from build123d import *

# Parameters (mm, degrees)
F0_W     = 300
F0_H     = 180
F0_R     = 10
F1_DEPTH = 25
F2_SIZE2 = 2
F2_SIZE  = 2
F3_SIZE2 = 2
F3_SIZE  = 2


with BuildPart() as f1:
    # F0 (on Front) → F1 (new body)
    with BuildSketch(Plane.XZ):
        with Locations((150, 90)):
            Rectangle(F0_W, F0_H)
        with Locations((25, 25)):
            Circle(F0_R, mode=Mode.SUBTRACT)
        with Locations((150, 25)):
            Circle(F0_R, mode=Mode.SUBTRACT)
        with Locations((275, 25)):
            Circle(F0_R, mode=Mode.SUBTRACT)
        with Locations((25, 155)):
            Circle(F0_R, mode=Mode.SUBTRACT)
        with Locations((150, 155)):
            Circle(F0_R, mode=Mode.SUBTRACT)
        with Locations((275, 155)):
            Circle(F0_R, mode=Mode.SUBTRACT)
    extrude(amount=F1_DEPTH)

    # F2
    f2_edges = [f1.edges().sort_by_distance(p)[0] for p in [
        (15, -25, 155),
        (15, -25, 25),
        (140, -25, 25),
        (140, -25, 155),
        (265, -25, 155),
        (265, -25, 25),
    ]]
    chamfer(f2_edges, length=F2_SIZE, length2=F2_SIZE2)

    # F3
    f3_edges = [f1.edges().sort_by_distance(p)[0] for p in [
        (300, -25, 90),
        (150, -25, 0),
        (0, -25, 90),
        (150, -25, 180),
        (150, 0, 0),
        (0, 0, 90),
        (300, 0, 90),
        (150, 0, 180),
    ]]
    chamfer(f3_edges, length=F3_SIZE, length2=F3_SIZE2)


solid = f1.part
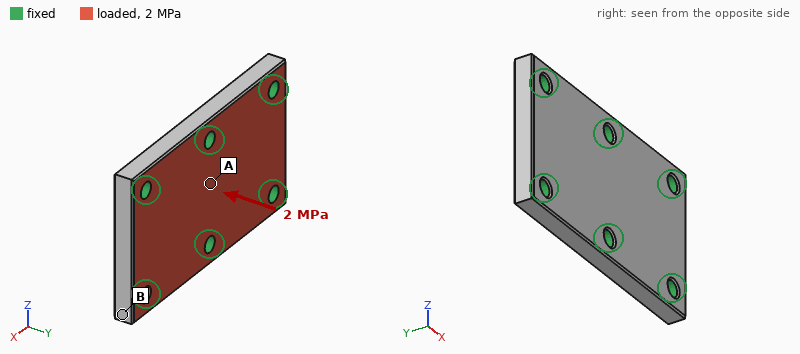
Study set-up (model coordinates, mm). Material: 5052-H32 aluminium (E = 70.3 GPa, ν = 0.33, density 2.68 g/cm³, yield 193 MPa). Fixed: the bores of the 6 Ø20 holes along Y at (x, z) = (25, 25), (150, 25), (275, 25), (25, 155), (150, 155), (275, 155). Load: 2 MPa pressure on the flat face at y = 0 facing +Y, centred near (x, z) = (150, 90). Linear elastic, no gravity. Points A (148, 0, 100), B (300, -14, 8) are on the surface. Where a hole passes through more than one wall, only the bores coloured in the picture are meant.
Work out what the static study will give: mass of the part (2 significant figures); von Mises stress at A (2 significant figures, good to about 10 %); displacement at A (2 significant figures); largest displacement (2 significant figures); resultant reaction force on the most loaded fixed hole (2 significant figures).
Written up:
3.5 kg
15 MPa
31 µm
39 µm
22 kN
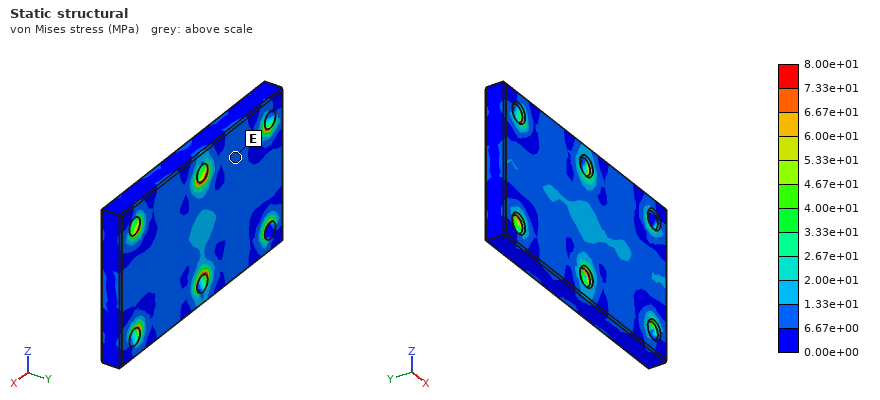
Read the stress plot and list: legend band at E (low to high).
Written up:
6.67e+00 to 1.33e+01 MPa
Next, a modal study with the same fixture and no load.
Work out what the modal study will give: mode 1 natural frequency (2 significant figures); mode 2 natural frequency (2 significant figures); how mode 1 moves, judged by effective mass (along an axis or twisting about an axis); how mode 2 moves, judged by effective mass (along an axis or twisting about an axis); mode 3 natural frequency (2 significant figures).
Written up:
5200 Hz
5500 Hz
along Y
twisting about Z
7700 Hz
